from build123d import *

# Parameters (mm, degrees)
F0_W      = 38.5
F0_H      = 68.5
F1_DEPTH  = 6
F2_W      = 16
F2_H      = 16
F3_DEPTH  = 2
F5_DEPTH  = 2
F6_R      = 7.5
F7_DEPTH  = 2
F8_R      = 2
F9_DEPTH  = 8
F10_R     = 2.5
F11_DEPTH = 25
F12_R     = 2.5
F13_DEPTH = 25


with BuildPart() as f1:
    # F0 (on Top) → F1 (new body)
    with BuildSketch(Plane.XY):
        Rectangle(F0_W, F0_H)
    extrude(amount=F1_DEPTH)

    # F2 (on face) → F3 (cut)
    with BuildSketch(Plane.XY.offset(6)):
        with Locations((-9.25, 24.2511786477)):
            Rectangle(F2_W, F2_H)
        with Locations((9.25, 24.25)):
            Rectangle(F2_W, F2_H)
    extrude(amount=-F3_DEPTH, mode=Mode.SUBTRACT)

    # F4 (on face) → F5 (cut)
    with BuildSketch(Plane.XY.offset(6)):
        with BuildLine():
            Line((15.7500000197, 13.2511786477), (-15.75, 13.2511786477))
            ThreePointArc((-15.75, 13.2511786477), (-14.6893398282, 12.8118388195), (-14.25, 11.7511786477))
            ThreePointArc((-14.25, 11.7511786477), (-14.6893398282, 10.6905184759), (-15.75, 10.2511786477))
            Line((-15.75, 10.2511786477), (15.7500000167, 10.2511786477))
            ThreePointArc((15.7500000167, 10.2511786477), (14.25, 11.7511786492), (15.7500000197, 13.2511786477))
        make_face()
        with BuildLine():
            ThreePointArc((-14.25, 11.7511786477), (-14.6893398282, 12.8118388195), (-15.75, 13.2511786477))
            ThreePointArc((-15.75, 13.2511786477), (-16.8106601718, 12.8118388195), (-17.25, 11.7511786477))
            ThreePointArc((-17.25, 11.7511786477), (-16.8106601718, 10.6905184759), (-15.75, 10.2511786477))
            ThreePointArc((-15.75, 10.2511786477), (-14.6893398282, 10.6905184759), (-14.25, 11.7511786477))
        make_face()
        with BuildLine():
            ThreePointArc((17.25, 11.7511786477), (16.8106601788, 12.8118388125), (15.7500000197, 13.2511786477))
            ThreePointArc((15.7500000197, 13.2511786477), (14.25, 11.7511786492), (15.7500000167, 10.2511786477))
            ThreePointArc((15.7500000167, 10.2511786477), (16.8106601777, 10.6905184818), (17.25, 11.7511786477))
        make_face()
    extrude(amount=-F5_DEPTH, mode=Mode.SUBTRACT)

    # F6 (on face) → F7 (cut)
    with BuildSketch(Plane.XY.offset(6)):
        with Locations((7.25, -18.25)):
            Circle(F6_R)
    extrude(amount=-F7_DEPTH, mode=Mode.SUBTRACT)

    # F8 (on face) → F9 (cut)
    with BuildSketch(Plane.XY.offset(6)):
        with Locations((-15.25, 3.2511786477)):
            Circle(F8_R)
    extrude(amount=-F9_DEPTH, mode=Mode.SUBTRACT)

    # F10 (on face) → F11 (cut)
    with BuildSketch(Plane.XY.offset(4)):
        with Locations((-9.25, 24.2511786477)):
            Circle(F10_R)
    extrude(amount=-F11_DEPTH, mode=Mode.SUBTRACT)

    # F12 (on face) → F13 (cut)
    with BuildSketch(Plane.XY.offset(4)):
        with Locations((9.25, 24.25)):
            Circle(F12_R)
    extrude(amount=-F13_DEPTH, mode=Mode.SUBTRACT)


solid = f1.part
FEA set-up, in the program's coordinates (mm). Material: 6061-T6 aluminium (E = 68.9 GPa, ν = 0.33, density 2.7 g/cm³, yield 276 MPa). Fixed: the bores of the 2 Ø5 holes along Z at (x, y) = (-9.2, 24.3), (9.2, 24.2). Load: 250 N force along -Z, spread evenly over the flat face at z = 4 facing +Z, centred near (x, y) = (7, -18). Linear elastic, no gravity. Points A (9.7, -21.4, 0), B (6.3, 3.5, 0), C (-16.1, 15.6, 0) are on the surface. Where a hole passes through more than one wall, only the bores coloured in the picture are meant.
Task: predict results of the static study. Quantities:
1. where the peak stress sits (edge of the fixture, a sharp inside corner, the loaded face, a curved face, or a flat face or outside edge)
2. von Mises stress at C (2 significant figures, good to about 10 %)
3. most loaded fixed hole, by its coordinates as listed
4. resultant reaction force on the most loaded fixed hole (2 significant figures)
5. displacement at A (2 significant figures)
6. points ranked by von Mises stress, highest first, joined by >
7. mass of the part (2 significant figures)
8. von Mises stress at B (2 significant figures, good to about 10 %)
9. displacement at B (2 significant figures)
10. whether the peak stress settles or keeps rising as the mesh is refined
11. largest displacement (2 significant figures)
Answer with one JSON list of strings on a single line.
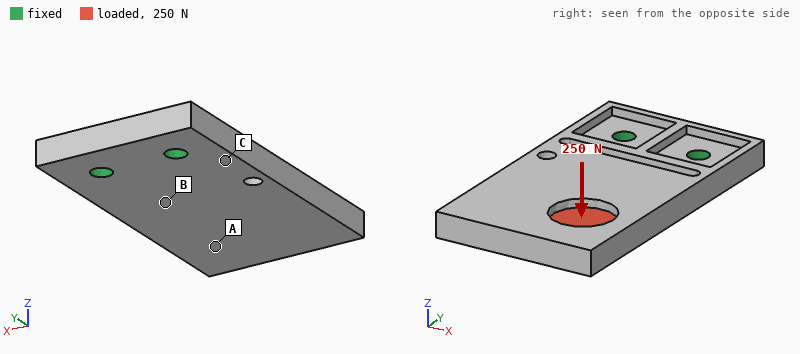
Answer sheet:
["edge of the fixture", "53 MPa", "(9.2, 24.2)", "210 N", "0.30 mm", "C > B > A", "38 g", "24 MPa", "0.096 mm", "keeps rising", "0.43 mm"]
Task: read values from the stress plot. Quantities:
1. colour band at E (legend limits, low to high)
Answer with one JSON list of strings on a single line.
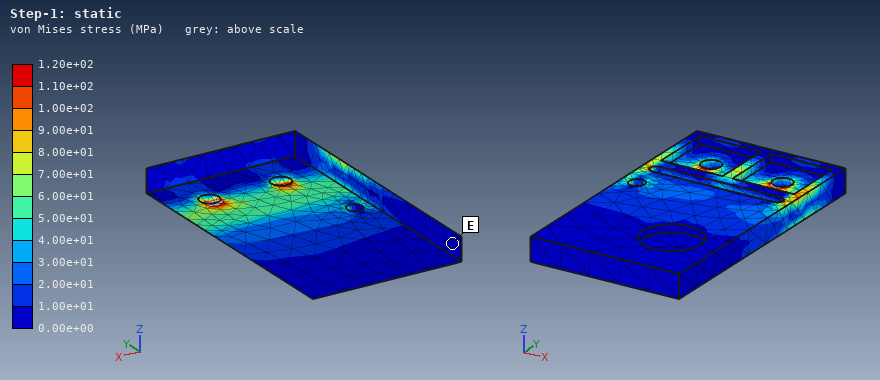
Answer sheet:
["0.00e+00 to 1.00e+01 MPa"]
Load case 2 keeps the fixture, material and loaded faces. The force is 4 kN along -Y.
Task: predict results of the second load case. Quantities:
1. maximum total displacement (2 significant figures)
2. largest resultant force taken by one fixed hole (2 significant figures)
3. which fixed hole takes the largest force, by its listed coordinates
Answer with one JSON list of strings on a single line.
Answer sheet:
["0.38 mm", "3.4 kN", "(9.2, 24.2)"]
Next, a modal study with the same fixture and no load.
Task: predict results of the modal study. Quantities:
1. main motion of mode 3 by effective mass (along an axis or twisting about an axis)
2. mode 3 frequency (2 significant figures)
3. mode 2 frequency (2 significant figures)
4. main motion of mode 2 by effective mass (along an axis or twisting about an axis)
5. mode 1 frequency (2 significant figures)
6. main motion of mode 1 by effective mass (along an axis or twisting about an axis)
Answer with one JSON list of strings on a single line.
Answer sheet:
["along X", "5600 Hz", "3800 Hz", "twisting about Y", "1000 Hz", "along Z"]
